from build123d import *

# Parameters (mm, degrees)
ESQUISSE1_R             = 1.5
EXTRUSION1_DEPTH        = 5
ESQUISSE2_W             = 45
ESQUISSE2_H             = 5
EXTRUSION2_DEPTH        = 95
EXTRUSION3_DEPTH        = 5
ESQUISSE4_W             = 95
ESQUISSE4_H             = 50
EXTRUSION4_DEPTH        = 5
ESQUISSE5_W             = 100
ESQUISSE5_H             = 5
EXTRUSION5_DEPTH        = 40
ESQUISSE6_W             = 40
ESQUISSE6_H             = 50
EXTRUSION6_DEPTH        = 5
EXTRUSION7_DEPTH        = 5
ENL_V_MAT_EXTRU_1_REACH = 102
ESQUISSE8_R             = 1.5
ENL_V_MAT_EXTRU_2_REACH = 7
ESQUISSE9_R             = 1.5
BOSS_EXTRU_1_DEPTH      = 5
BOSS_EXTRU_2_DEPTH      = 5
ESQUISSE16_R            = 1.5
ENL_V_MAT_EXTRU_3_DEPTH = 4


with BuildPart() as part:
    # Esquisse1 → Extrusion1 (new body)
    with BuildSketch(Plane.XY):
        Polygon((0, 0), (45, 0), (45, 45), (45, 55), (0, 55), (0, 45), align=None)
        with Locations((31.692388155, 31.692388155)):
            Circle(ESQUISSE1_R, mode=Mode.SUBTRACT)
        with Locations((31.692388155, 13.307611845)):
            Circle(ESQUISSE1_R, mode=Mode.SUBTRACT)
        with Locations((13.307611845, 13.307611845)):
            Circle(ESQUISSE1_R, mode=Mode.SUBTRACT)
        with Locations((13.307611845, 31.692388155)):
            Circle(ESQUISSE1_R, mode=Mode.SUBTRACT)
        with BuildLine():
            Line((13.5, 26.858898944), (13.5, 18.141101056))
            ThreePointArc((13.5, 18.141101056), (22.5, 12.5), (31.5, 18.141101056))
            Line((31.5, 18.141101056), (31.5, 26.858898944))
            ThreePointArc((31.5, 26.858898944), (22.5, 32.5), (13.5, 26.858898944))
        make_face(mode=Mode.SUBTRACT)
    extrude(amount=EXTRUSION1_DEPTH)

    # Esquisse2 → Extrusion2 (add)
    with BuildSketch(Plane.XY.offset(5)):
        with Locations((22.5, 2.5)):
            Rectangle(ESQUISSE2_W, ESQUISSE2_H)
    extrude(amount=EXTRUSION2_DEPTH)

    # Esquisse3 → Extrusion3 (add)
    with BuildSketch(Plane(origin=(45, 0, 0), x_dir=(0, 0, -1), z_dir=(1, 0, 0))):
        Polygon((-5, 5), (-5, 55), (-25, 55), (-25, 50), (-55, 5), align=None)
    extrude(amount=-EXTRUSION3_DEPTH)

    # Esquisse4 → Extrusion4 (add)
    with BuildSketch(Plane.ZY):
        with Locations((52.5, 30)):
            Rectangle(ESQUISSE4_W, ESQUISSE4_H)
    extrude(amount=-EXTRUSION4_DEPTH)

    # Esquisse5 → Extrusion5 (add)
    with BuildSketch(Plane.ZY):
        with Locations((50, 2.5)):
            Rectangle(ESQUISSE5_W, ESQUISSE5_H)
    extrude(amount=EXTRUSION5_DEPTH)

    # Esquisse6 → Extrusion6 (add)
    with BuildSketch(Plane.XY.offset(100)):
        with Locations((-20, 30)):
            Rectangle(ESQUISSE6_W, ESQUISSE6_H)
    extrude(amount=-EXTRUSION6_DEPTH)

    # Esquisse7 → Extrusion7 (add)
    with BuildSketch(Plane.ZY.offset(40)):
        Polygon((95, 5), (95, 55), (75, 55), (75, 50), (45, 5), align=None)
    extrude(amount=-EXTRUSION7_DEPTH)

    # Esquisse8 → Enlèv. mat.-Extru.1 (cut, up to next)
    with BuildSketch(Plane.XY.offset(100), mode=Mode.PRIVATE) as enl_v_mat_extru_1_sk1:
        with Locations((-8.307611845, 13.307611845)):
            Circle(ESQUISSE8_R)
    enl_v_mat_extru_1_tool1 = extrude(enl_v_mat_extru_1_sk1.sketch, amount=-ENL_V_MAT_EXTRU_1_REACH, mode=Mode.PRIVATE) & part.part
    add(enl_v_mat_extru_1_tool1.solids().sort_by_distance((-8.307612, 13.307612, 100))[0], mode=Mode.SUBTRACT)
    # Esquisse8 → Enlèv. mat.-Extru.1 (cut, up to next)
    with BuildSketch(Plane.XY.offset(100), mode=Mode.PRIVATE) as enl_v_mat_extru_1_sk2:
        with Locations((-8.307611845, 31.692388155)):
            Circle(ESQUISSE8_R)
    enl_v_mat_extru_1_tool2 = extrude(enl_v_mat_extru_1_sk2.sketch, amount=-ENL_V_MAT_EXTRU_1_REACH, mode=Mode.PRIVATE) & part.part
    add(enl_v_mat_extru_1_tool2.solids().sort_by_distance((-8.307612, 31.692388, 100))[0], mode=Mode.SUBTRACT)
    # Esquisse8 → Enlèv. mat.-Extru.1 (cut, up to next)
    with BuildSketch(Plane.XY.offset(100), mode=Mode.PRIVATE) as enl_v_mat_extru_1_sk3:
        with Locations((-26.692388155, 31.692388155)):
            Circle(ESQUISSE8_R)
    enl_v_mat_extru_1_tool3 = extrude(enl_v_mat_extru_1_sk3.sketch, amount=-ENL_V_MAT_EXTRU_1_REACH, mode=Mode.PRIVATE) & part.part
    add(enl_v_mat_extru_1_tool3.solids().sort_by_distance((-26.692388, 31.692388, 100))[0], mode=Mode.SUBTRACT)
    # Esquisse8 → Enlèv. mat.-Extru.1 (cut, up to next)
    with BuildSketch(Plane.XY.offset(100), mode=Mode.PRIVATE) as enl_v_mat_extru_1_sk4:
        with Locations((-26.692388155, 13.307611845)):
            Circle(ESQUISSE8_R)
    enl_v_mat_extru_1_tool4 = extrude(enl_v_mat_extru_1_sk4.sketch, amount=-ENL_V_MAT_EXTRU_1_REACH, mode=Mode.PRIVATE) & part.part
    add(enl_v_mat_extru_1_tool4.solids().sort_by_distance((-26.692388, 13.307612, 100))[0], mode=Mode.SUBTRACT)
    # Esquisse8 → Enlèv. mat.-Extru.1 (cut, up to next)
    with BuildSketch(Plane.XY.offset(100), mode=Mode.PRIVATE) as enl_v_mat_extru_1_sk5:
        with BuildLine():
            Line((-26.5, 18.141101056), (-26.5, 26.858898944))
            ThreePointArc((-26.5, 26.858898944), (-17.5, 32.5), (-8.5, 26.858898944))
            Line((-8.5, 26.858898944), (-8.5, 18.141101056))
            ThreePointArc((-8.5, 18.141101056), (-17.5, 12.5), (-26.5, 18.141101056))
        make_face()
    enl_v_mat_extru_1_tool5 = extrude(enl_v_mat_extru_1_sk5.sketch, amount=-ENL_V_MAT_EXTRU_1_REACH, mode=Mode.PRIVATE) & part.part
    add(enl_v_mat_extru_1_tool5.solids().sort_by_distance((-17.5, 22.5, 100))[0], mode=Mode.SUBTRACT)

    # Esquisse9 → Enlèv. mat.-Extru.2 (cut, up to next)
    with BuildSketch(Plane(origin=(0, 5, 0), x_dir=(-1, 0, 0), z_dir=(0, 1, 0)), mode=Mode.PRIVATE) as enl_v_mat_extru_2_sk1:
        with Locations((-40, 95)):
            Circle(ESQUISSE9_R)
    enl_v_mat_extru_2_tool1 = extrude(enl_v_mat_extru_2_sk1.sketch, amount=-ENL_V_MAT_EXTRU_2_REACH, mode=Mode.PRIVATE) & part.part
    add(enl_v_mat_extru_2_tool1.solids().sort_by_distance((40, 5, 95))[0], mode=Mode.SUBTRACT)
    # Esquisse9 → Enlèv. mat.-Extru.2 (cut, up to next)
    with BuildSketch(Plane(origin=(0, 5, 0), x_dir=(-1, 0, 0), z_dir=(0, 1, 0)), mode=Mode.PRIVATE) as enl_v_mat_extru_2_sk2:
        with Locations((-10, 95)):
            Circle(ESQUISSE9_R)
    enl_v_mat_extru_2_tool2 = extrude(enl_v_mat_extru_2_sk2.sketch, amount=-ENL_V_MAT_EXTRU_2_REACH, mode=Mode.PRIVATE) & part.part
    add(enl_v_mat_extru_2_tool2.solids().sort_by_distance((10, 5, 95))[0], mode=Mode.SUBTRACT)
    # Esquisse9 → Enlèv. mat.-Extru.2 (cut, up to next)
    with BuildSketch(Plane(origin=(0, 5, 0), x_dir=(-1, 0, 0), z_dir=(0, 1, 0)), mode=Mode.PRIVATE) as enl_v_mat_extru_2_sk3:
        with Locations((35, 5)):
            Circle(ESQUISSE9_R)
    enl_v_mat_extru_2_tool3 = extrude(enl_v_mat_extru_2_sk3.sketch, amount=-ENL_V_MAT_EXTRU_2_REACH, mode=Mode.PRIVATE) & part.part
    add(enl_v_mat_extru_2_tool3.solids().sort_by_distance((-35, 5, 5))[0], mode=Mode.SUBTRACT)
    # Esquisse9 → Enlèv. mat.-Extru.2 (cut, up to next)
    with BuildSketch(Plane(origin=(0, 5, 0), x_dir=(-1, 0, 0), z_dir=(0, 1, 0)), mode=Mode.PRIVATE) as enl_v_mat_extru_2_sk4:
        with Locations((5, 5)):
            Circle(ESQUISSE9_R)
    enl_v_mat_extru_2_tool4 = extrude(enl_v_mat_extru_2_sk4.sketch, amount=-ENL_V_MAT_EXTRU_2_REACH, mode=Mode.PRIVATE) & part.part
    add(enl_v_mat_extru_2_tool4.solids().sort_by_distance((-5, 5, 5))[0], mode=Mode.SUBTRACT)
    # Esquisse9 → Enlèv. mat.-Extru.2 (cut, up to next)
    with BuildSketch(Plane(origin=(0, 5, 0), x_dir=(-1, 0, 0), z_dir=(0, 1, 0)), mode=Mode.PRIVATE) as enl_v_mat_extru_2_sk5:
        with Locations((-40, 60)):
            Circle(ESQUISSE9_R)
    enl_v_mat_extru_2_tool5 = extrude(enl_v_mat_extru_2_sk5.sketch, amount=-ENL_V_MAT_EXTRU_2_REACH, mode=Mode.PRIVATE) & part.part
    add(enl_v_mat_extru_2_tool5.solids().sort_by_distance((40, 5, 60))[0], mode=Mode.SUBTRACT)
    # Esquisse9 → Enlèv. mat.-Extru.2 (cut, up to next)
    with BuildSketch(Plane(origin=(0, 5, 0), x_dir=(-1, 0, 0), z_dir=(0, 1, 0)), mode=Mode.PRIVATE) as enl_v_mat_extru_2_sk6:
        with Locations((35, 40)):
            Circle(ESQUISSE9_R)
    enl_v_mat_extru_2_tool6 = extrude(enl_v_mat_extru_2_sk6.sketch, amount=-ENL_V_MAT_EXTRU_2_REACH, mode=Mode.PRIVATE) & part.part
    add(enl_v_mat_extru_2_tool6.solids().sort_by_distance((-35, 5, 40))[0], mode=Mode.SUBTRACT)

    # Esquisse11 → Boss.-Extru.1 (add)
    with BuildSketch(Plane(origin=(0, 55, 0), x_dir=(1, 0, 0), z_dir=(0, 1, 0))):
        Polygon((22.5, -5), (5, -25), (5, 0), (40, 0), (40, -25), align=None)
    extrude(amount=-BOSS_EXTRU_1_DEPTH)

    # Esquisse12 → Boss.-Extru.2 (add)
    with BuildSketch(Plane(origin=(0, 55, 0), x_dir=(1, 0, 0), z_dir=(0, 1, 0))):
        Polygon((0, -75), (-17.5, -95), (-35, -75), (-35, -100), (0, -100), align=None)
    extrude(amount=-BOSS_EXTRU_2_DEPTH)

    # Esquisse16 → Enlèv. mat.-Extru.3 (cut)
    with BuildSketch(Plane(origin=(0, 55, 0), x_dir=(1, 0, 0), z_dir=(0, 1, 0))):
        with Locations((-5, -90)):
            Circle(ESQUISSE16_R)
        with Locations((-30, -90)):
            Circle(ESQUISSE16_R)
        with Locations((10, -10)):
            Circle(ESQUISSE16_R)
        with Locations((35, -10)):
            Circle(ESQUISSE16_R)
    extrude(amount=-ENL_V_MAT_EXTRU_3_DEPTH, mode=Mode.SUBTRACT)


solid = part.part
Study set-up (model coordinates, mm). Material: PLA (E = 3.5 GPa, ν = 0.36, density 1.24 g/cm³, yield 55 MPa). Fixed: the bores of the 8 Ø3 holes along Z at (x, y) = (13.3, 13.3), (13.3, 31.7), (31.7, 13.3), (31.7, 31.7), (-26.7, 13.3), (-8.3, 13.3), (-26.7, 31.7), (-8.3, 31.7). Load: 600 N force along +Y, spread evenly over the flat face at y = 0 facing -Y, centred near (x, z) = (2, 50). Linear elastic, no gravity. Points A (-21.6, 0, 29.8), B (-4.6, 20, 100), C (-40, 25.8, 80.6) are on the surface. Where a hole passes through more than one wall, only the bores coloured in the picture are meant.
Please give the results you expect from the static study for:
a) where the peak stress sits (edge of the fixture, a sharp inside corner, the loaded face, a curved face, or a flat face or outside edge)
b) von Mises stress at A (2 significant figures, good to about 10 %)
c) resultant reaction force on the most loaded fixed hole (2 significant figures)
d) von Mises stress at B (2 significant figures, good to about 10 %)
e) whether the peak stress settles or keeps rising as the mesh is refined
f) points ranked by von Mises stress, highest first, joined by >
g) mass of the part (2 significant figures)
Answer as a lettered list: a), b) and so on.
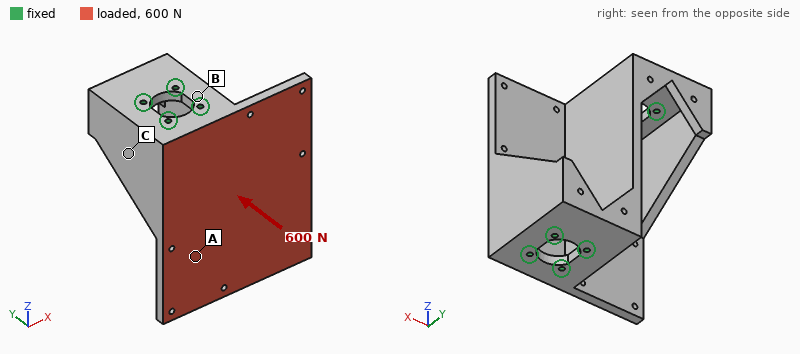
a) edge of the fixture
b) 3.4 MPa
c) 120 N
d) 1.7 MPa
e) keeps rising
f) A > B > C
g) 130 g
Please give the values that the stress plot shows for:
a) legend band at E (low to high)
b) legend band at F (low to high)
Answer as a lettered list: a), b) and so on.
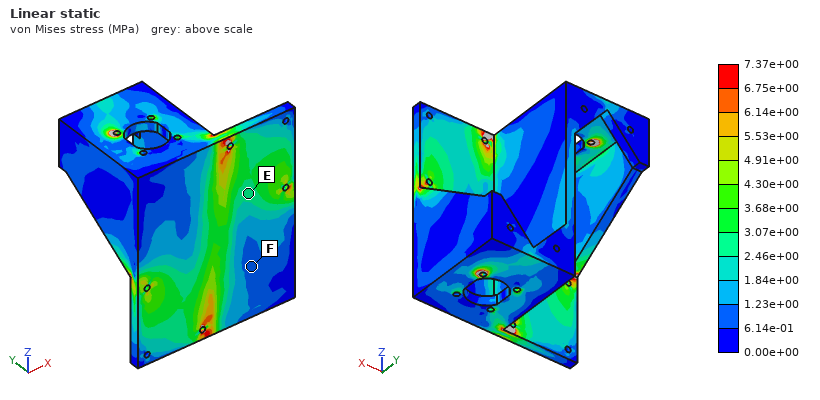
a) 2.46e+00 to 3.07e+00 MPa
b) 6.14e-01 to 1.23e+00 MPa
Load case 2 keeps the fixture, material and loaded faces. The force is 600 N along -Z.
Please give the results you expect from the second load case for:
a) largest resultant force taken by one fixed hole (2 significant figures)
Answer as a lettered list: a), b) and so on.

a) 150 N
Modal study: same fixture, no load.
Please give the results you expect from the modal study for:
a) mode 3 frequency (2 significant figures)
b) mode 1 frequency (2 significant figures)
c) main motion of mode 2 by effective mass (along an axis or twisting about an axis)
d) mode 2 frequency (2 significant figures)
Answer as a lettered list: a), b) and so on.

a) 1400 Hz
b) 1000 Hz
c) along Y
d) 1100 Hz
